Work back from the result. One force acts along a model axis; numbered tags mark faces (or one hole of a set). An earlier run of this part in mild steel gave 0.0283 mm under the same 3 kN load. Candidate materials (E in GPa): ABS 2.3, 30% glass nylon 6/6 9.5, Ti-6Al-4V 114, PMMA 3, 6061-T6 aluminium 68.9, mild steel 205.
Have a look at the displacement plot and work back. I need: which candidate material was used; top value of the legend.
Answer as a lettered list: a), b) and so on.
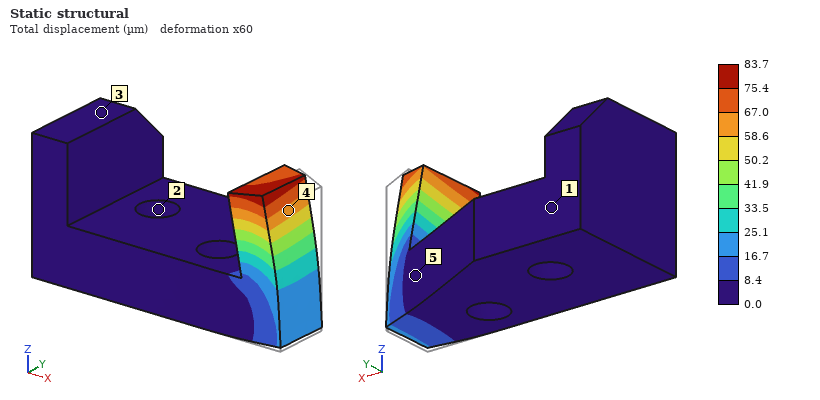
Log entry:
a) 6061-T6 aluminium
b) 83.7 µm
